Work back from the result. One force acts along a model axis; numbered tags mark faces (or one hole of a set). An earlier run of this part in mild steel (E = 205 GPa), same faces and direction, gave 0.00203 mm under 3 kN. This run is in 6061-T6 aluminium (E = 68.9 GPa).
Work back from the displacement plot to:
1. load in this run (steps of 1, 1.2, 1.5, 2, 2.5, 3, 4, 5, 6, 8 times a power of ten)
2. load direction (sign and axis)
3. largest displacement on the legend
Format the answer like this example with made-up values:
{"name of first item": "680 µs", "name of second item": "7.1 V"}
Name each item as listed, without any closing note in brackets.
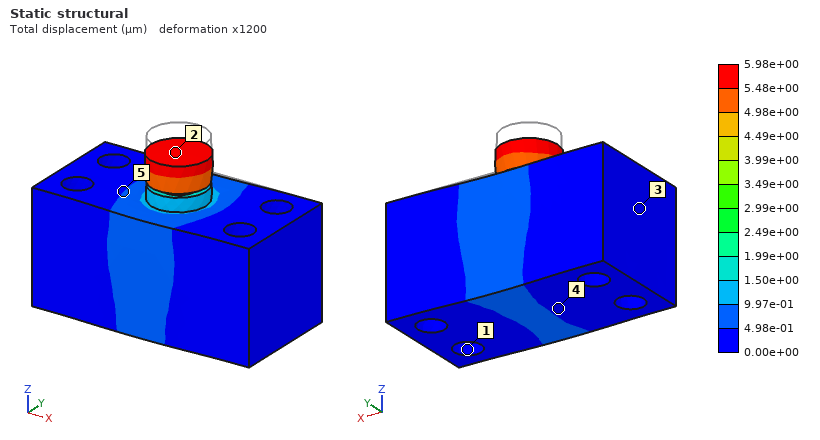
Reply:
{"load in this run": "3 kN", "load direction": "-Z", "largest displacement on the legend": "5.98e+00 µm"}
